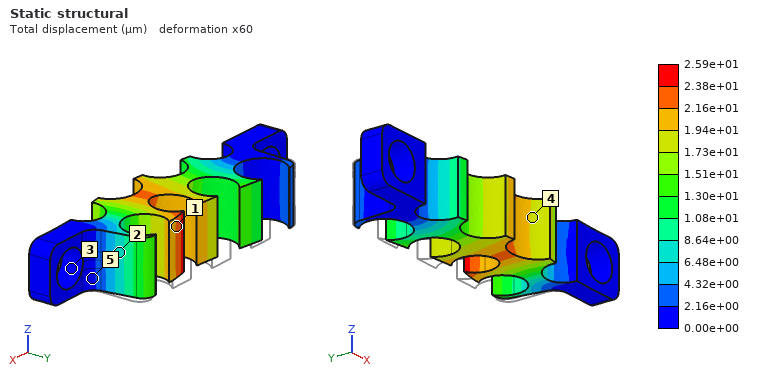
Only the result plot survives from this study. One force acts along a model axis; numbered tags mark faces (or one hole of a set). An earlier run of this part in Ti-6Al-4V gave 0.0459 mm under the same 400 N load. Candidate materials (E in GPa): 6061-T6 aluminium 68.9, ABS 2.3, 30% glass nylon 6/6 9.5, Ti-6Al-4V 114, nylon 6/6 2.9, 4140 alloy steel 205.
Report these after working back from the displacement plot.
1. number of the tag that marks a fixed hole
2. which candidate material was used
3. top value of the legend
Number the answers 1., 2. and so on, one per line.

1. 3
2. 4140 alloy steel
3. 2.59e+01 µm
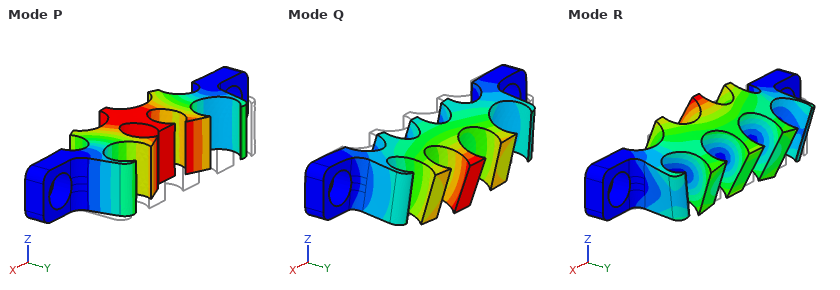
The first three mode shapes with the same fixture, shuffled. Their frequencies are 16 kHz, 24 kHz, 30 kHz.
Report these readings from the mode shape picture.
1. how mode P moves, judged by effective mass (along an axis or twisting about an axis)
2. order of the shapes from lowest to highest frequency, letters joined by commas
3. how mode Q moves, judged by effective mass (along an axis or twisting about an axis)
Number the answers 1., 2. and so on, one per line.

1. along Y
2. P, Q, R
3. along Z
